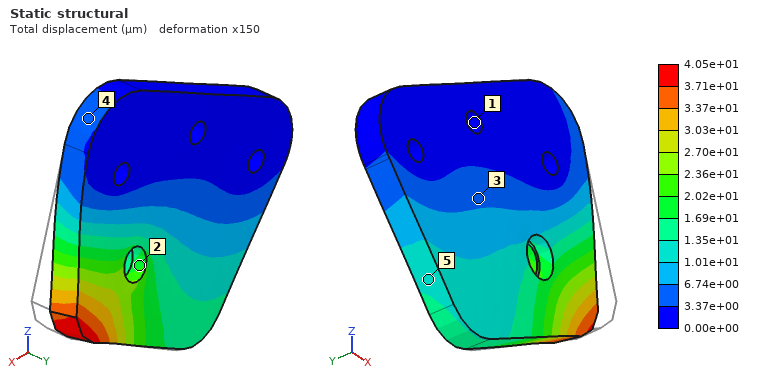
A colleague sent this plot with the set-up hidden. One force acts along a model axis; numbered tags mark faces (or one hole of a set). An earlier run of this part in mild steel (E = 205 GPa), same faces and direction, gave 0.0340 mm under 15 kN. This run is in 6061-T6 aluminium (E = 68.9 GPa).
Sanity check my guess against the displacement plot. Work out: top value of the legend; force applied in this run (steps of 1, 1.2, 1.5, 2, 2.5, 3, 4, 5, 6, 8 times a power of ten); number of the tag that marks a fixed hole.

4.05e+01 µm
6 kN
1
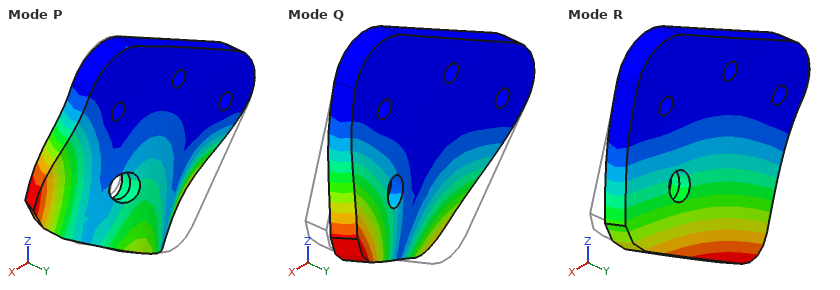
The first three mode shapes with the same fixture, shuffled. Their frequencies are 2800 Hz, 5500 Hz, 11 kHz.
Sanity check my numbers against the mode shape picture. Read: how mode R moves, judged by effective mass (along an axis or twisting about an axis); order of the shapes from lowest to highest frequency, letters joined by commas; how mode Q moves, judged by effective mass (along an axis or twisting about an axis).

along Y
R, Q, P
twisting about Z
